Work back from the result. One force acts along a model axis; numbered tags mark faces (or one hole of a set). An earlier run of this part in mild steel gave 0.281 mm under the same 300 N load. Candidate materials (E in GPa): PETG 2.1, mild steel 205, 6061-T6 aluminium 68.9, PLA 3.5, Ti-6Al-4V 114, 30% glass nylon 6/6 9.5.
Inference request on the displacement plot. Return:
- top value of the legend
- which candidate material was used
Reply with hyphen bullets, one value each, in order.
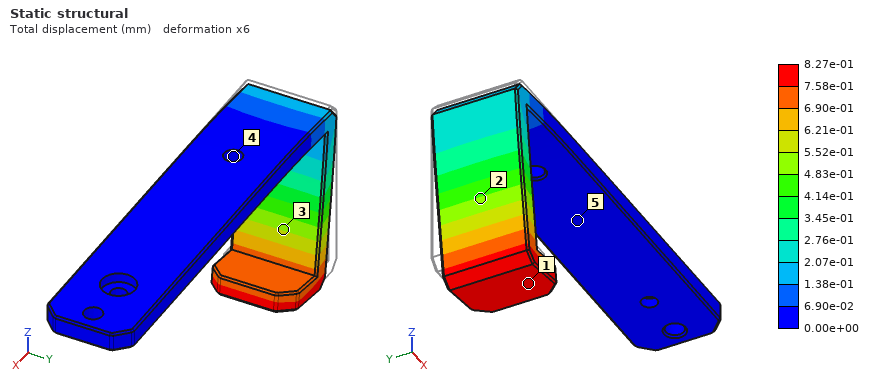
- 8.27e-01 mm
- 6061-T6 aluminium
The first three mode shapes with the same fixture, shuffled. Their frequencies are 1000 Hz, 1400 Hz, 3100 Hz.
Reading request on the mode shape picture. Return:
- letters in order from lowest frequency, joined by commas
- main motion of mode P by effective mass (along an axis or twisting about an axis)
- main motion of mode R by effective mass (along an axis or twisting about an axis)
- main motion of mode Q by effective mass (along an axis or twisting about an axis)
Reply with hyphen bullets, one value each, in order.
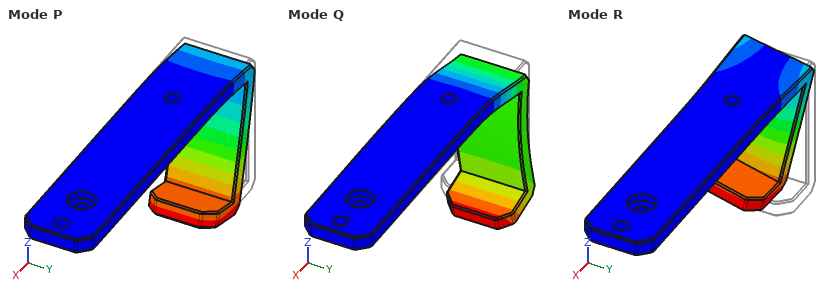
- P, R, Q
- along X
- along Y
- along Z
